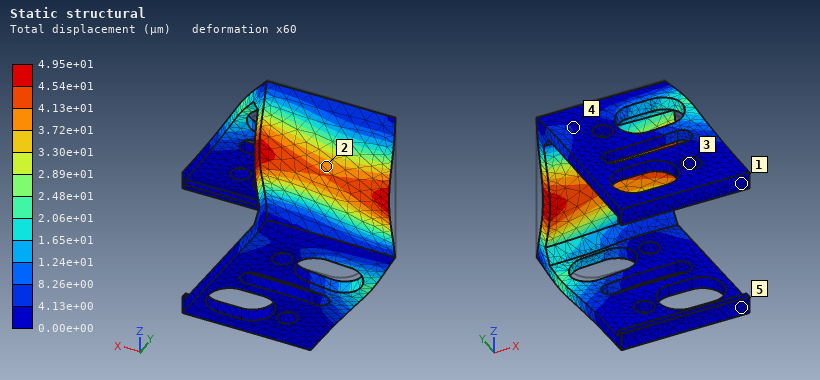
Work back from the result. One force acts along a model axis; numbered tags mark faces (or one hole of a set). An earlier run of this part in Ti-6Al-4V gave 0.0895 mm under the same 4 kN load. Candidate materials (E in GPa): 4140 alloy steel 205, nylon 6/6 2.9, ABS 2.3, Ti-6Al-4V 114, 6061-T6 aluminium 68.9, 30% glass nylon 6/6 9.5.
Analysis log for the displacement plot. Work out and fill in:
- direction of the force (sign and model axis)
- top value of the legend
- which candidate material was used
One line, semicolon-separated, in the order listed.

-Y; 4.95e+01 µm; 4140 alloy steel
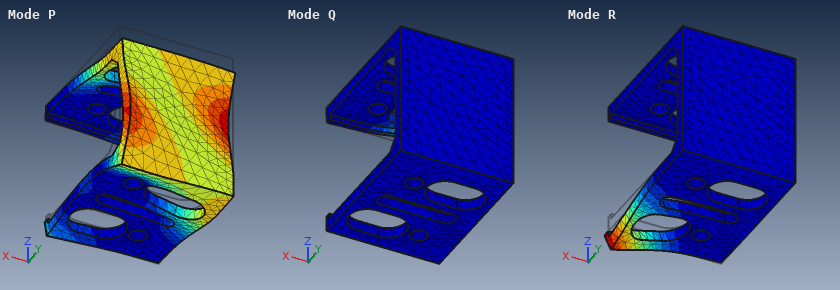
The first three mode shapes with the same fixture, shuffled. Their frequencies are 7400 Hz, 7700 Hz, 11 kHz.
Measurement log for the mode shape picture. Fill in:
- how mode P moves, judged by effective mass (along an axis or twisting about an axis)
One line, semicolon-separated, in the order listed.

along Z
